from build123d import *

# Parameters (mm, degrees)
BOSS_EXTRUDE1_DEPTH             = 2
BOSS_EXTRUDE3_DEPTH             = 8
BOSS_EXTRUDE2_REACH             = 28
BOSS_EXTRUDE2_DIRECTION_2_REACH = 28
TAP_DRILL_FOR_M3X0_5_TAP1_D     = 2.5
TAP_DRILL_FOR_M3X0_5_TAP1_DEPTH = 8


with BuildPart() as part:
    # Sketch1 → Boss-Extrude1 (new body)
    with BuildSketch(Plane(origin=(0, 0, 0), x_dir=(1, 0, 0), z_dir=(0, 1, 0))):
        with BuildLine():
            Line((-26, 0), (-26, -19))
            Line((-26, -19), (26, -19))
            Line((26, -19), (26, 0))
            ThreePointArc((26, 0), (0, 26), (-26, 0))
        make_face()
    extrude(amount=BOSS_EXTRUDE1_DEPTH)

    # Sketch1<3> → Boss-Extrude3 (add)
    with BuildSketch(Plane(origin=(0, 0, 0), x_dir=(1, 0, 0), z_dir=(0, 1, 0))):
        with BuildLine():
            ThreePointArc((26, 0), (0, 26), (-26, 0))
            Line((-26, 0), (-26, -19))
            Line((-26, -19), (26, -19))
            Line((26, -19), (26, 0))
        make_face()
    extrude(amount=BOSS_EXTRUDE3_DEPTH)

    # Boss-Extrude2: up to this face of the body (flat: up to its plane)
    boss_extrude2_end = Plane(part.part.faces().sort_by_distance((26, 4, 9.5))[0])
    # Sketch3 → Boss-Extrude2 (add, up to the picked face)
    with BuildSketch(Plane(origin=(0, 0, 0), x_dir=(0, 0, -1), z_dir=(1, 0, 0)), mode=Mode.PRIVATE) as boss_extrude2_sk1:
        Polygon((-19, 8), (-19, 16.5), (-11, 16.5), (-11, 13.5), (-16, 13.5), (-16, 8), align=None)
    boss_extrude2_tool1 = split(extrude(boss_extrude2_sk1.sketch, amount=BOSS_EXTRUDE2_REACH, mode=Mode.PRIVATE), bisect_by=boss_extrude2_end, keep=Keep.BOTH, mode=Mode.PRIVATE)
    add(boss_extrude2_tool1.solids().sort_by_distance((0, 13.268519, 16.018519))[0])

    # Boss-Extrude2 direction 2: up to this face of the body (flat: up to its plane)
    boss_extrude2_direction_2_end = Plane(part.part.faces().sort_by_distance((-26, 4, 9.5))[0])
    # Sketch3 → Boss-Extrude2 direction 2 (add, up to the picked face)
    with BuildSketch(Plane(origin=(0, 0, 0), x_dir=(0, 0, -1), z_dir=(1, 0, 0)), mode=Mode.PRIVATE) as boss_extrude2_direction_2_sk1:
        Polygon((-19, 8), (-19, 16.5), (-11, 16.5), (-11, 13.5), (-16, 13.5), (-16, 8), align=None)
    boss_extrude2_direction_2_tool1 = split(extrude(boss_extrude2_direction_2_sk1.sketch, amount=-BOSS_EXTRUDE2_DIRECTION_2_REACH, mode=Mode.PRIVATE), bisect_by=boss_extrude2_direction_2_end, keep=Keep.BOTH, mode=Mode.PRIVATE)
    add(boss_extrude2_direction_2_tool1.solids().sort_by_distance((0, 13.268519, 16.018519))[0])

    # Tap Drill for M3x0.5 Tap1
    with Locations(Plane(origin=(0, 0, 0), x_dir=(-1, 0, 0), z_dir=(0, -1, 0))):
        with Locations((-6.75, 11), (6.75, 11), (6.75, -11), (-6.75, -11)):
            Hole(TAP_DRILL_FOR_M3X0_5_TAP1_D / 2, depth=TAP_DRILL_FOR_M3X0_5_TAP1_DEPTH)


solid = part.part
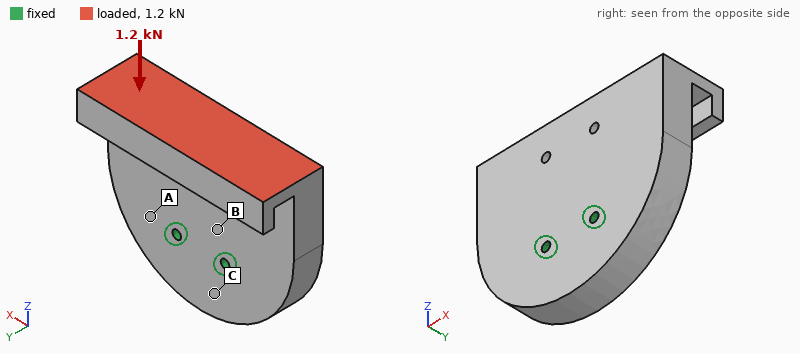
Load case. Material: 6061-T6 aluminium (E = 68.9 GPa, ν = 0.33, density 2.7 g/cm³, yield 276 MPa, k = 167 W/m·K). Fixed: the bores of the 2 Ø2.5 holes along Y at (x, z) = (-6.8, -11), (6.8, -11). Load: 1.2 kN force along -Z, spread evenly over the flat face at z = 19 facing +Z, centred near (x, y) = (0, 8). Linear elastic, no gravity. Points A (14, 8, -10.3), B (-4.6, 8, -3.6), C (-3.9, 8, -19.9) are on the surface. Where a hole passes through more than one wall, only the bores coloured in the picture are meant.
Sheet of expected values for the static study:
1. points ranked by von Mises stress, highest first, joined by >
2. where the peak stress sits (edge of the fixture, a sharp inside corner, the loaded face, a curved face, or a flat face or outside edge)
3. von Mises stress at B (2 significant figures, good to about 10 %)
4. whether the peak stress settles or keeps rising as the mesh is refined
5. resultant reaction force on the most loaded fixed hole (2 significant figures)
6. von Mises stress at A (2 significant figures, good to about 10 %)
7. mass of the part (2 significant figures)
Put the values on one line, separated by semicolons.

B > A > C; edge of the fixture; 15 MPa; keeps rising; 600 N; 8.2 MPa; 50 g
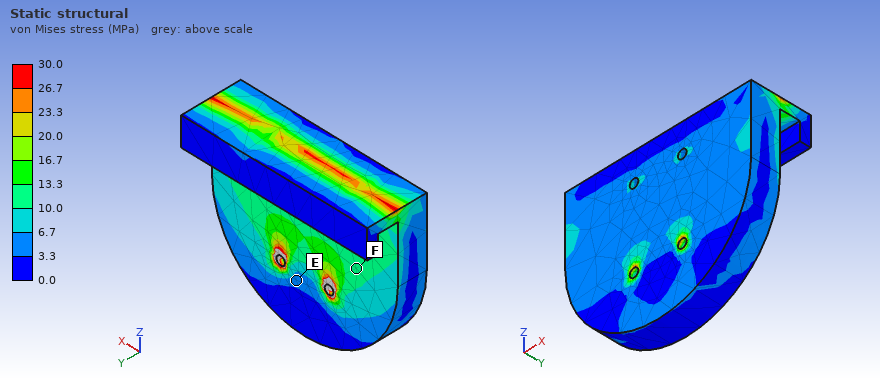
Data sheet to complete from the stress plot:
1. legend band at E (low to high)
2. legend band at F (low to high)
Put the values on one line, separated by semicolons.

3.3 to 6.7 MPa; 10.0 to 13.3 MPa
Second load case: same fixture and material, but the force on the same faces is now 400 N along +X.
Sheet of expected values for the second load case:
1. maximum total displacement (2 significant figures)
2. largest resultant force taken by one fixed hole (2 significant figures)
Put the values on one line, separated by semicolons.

12 µm; 820 N
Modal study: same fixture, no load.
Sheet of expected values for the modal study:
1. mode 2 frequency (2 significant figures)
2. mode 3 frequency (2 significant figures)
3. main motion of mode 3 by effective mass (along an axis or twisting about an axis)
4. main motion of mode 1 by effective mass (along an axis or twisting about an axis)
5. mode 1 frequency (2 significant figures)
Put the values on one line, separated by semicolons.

6000 Hz; 8200 Hz; along X; along Y; 4200 Hz
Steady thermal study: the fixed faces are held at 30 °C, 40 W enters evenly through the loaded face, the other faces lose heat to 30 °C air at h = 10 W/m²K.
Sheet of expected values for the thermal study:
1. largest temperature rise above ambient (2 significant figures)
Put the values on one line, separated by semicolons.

25 K
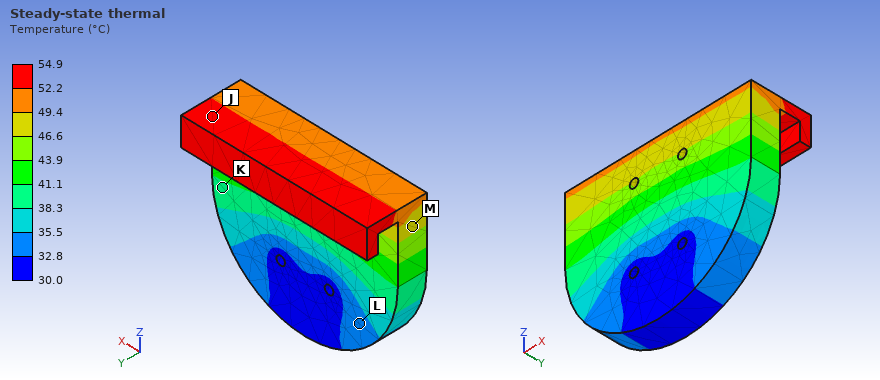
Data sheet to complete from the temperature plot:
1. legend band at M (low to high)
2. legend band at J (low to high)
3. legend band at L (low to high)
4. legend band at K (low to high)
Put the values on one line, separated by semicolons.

46.6 to 49.4 °C; 52.2 to 54.9 °C; 32.8 to 35.5 °C; 38.3 to 41.1 °C
